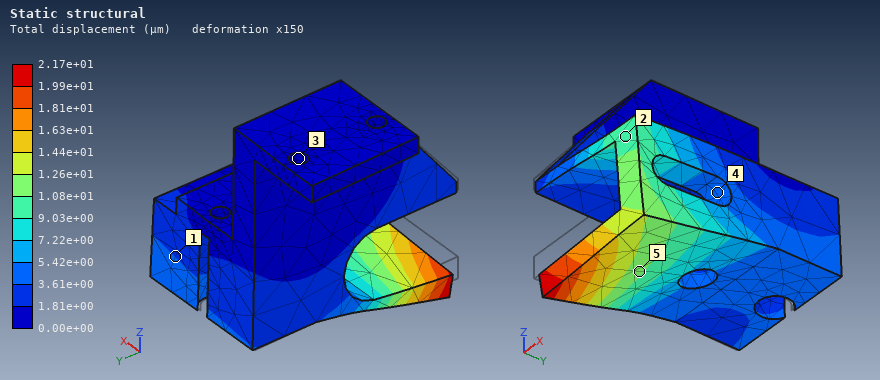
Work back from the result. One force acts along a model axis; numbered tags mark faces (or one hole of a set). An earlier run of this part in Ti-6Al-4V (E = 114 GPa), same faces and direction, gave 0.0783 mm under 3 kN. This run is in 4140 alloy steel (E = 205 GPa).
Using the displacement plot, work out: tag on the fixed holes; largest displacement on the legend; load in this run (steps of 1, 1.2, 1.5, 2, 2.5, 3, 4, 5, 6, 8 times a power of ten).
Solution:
3
2.17e+01 µm
1.5 kN
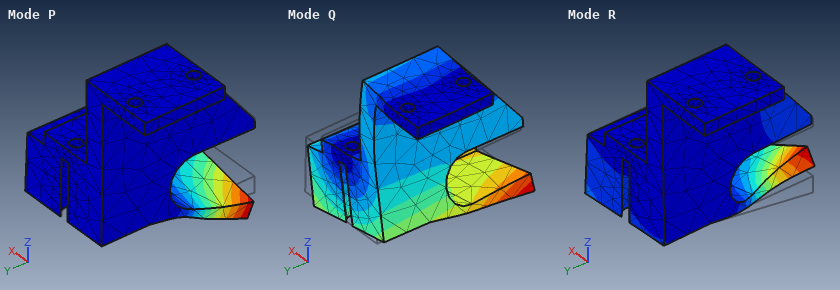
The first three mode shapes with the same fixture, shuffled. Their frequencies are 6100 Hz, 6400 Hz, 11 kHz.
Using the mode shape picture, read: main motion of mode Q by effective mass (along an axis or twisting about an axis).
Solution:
along X
